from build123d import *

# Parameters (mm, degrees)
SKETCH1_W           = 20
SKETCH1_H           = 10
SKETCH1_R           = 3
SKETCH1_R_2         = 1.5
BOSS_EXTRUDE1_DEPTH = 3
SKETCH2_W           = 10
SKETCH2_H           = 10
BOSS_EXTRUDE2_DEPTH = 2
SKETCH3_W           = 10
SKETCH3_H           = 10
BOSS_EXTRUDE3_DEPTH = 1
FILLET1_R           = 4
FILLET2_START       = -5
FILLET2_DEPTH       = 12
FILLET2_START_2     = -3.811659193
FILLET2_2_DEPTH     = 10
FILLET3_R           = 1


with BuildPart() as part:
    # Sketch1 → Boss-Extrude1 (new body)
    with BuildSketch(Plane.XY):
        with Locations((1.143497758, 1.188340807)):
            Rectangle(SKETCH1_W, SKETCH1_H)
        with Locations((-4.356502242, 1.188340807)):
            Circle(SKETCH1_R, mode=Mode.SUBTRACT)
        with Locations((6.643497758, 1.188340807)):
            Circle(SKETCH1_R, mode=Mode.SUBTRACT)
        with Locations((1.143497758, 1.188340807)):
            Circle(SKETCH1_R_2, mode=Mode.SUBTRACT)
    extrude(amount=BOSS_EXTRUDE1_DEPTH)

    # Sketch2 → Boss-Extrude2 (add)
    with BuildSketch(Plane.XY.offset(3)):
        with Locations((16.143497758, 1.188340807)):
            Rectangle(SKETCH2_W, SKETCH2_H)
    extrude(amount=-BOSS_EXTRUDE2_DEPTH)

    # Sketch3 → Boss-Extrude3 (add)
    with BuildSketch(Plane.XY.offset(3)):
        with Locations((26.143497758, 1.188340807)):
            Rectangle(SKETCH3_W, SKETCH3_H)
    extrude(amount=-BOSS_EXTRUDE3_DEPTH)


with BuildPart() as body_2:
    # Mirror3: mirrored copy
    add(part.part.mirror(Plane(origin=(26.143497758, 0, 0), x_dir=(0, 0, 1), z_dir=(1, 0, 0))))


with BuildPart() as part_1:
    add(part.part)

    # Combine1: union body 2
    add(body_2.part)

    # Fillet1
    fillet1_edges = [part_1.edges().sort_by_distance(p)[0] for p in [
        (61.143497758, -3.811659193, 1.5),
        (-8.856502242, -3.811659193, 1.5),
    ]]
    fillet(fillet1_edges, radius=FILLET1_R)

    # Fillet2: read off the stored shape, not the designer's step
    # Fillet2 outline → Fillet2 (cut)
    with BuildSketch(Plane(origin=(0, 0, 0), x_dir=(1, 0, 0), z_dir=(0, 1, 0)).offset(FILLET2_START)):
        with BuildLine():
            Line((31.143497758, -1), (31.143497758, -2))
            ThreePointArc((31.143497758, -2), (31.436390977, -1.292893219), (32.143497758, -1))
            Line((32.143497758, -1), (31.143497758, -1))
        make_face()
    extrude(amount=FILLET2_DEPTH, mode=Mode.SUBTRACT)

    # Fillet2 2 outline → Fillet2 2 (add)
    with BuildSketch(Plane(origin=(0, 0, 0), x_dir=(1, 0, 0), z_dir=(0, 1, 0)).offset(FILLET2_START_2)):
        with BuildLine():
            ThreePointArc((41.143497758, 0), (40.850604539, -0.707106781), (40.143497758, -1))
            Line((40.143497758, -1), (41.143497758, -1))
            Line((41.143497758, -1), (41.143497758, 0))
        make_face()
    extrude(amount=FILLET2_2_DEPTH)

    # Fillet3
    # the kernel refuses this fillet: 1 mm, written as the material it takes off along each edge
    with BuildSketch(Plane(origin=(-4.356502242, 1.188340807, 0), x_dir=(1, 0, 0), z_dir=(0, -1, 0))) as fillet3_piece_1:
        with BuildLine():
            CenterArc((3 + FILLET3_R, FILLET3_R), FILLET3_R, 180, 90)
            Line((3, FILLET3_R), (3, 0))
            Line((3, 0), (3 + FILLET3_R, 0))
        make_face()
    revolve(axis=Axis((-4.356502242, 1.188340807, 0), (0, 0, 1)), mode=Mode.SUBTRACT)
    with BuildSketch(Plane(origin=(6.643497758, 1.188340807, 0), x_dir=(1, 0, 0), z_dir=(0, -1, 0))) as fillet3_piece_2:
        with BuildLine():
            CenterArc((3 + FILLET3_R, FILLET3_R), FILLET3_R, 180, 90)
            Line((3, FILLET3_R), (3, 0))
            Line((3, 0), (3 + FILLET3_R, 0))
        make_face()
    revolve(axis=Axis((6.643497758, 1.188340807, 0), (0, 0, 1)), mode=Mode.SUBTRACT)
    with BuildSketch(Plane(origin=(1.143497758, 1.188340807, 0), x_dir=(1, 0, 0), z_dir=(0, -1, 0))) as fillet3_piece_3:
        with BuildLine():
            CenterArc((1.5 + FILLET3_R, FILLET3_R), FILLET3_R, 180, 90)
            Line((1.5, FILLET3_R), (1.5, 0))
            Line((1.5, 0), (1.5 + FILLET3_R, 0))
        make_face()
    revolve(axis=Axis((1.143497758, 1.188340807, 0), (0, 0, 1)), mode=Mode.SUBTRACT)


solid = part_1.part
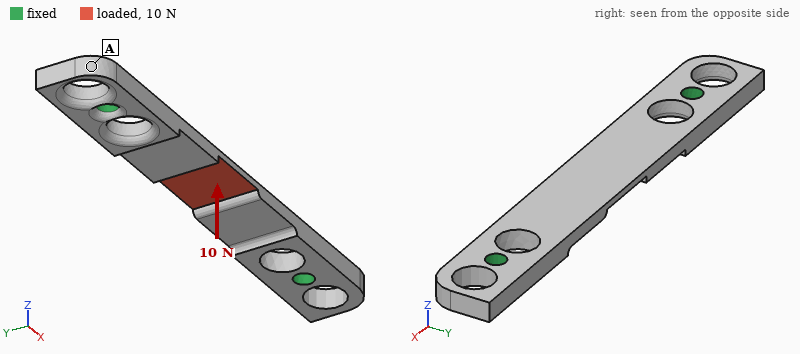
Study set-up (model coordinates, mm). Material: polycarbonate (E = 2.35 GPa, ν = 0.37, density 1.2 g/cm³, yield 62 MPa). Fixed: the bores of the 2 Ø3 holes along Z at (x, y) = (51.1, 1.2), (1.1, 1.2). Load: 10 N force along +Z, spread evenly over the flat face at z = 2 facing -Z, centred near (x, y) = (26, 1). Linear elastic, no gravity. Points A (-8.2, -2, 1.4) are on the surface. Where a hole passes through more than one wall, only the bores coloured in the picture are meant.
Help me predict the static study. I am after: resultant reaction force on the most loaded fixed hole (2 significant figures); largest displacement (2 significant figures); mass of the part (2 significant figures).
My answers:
25 N
0.46 mm
1.5 g
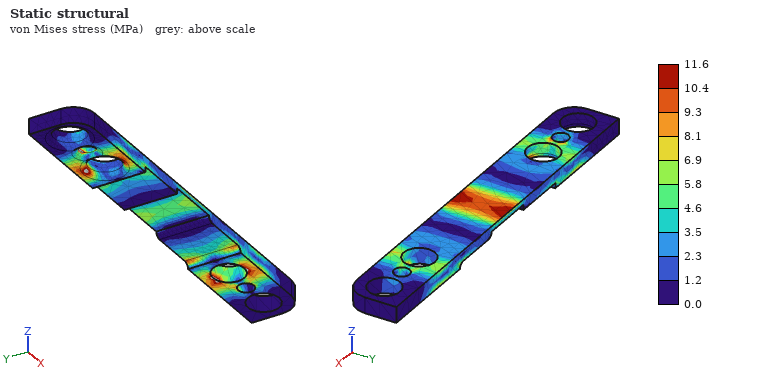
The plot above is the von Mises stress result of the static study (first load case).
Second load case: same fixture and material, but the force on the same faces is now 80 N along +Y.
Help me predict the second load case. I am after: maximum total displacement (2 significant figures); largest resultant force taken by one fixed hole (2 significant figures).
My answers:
0.39 mm
41 N
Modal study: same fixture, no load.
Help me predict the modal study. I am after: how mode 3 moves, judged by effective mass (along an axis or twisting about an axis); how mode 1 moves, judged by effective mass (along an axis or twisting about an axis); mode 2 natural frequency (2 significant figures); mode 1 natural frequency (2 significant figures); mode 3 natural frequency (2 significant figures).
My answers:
along Y
along Z
2800 Hz
1400 Hz
3300 Hz
